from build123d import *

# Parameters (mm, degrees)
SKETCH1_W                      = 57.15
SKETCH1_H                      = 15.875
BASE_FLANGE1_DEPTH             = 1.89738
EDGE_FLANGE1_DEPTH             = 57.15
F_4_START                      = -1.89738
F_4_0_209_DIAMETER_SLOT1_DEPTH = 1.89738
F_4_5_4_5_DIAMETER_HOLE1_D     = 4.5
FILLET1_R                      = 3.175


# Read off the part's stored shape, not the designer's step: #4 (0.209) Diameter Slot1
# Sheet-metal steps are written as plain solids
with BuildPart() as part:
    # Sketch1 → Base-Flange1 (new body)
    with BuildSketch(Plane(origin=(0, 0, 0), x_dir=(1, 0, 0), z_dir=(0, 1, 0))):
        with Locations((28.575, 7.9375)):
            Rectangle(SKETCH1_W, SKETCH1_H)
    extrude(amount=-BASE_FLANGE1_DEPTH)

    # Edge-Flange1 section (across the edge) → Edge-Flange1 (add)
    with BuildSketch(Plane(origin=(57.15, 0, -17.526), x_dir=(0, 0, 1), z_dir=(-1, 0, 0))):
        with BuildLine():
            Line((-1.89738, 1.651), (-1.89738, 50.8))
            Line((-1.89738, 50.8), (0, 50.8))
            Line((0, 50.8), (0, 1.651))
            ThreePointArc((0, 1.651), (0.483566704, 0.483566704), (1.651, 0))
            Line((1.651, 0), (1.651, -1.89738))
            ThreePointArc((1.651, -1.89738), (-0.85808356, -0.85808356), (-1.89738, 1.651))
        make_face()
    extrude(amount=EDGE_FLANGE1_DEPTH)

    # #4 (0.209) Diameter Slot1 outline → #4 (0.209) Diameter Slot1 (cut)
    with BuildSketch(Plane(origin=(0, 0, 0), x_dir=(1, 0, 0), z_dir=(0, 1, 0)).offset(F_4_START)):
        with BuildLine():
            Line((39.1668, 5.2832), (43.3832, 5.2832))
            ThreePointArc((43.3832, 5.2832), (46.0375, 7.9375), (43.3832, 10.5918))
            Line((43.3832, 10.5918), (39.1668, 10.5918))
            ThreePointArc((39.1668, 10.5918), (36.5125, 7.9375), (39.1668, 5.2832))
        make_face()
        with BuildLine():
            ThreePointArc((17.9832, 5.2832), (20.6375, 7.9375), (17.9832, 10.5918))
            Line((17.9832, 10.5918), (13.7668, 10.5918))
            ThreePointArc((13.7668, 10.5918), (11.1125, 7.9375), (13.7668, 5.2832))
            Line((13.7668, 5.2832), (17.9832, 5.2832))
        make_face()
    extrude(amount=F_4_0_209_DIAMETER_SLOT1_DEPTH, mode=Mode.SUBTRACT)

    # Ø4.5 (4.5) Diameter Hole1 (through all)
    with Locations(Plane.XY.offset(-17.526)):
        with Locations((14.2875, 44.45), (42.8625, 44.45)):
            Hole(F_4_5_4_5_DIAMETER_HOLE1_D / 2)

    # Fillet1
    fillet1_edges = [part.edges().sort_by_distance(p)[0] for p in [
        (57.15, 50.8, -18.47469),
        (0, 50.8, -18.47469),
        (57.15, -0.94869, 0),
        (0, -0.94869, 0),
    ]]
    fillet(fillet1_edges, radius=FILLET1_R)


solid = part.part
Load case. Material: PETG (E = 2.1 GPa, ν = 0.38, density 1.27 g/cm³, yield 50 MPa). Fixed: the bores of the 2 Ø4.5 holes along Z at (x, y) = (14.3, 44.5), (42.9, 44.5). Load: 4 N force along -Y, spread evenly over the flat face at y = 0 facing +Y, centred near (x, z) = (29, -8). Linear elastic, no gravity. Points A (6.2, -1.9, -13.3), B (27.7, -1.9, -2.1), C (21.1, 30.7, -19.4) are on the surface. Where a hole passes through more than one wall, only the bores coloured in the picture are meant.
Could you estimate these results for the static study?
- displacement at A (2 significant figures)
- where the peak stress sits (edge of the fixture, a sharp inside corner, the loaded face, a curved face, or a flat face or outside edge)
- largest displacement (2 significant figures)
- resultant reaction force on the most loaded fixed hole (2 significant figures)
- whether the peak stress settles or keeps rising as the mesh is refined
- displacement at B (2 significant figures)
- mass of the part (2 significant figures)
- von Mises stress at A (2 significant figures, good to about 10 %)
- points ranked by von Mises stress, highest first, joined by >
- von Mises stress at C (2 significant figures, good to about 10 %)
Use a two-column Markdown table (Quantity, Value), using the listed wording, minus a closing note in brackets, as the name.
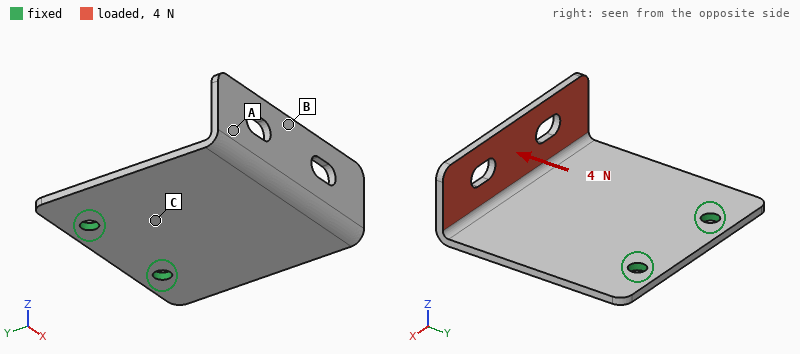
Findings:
| Quantity | Value |
|---|---|
| displacement at A | 0.63 mm |
| where the peak stress sits | edge of the fixture |
| largest displacement | 0.81 mm |
| resultant reaction force on the most loaded fixed hole | 2.0 N |
| whether the peak stress settles or keeps rising as the mesh is refined | keeps rising |
| displacement at B | 0.77 mm |
| mass of the part | 9.2 g |
| von Mises stress at A | 0.58 MPa |
| points ranked by von Mises stress, highest first, joined by > | C > A > B |
| von Mises stress at C | 1.0 MPa |
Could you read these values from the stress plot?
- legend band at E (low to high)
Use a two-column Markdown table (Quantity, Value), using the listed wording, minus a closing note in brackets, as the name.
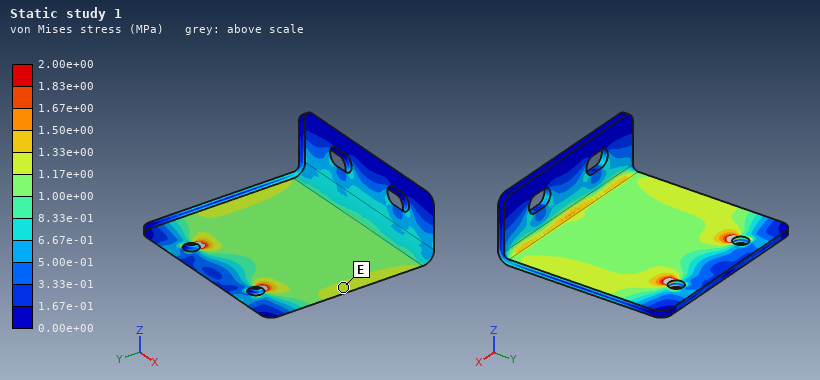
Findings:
| Quantity | Value |
|---|---|
| legend band at E | 1.17e+00 to 1.33e+00 MPa |
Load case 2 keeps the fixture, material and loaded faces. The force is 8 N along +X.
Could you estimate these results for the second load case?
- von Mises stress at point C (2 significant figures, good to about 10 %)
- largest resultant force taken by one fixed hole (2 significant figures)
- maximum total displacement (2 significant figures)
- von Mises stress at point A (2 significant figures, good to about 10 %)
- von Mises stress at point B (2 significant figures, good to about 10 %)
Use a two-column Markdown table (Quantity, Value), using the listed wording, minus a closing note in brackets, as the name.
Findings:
| Quantity | Value |
|---|---|
| von Mises stress at point C | 1.3 MPa |
| largest resultant force taken by one fixed hole | 12 N |
| maximum total displacement | 0.81 mm |
| von Mises stress at point A | 0.97 MPa |
| von Mises stress at point B | 0.79 MPa |
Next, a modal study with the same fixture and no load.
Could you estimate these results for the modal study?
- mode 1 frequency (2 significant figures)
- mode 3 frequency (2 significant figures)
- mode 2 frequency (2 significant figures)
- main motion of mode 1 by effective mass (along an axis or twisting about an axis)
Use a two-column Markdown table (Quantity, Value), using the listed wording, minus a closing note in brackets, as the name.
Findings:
| Quantity | Value |
|---|---|
| mode 1 frequency | 120 Hz |
| mode 3 frequency | 590 Hz |
| mode 2 frequency | 250 Hz |
| main motion of mode 1 by effective mass | along Z |
